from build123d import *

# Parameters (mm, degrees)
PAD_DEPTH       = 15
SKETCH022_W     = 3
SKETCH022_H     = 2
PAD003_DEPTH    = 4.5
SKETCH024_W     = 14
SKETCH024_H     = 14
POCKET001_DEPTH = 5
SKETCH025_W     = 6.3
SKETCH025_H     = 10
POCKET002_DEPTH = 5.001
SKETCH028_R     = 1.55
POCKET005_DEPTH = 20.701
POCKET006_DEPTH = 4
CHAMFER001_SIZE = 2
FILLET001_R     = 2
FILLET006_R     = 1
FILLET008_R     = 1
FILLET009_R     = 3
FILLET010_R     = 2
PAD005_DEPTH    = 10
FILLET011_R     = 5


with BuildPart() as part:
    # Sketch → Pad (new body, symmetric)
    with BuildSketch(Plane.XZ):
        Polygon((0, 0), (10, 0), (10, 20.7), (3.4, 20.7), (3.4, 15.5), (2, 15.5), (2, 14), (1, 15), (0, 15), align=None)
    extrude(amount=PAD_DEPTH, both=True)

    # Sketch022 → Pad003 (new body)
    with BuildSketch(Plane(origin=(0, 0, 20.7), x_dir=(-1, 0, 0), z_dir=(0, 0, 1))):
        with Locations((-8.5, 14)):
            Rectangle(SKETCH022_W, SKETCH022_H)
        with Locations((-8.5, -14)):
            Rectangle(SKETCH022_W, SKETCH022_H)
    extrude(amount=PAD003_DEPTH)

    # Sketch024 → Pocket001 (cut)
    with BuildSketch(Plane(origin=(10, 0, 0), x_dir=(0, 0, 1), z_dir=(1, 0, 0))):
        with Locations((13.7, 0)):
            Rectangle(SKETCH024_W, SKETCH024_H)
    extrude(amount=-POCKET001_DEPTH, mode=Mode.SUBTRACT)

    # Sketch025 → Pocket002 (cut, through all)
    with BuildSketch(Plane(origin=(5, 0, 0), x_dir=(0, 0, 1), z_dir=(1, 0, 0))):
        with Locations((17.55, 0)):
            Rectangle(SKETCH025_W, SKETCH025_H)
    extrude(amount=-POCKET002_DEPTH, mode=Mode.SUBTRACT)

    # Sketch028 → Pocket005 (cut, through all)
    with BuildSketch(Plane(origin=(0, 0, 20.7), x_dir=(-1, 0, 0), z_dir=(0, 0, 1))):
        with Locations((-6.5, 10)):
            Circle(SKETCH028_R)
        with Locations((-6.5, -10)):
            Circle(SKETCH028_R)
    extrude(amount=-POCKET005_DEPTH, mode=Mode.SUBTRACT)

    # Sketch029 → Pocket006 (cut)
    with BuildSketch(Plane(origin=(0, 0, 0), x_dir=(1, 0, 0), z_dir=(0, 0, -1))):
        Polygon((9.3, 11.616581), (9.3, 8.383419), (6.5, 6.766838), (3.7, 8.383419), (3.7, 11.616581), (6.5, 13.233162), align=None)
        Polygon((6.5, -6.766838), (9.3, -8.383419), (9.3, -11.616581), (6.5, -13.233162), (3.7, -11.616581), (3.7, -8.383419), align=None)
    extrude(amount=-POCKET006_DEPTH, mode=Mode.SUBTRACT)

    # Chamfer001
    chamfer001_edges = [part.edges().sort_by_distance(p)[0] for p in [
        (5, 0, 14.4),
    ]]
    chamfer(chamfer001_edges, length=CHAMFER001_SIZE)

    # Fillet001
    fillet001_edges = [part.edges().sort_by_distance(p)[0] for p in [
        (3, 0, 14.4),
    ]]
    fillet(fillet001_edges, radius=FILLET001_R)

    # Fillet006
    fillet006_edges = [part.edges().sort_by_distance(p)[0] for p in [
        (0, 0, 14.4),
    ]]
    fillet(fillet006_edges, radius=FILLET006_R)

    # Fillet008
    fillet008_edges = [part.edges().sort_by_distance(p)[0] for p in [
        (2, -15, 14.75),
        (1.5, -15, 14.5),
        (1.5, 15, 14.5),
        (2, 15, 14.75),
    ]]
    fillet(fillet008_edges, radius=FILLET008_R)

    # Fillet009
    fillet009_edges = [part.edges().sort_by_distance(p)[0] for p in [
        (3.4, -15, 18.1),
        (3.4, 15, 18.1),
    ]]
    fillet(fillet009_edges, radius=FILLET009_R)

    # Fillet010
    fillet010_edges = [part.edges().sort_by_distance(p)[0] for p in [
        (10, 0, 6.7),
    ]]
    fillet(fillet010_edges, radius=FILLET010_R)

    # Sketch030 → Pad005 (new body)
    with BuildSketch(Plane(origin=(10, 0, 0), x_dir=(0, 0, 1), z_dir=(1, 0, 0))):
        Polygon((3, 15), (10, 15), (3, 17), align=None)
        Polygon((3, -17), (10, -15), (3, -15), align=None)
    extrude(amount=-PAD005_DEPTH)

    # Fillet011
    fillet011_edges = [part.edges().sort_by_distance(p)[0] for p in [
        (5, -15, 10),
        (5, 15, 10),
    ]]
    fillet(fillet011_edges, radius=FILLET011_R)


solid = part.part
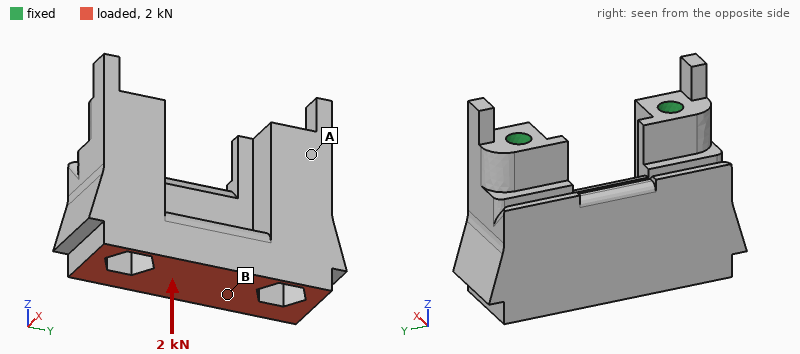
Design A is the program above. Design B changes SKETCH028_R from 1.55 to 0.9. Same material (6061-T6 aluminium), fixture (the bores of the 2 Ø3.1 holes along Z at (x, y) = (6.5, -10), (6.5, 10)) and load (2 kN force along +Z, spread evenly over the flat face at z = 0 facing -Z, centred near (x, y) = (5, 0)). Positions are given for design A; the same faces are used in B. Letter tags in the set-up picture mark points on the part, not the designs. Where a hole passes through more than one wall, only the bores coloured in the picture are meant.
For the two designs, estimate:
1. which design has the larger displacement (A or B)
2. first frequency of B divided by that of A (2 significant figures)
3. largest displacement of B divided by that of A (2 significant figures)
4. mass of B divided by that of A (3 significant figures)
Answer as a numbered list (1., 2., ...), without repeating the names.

1. B
2. 0.88
3. 1.1
4. 1.04
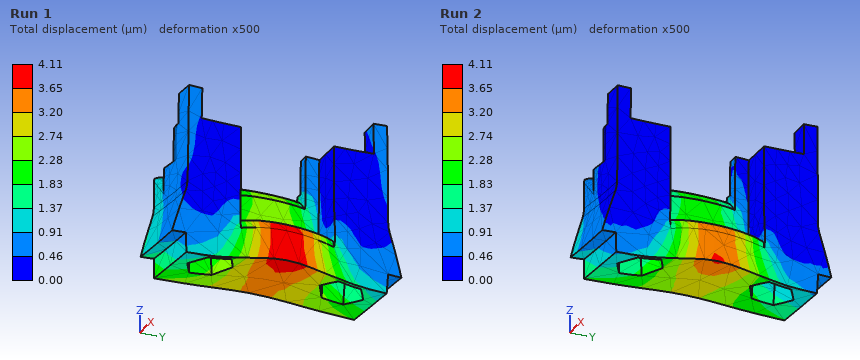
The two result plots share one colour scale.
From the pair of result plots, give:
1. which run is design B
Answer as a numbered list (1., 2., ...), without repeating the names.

1. Run 1
